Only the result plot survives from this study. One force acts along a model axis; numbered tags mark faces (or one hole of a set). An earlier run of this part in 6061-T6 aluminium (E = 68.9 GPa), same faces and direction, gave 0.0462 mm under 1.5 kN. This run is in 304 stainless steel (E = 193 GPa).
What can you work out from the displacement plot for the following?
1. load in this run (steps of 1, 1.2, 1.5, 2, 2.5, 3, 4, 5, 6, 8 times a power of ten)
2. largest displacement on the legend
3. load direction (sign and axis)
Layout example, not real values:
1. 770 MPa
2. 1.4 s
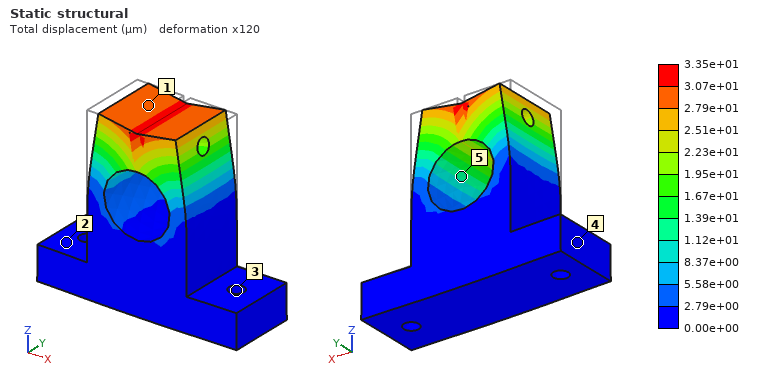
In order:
1. 3 kN
2. 3.35e+01 µm
3. -Z
